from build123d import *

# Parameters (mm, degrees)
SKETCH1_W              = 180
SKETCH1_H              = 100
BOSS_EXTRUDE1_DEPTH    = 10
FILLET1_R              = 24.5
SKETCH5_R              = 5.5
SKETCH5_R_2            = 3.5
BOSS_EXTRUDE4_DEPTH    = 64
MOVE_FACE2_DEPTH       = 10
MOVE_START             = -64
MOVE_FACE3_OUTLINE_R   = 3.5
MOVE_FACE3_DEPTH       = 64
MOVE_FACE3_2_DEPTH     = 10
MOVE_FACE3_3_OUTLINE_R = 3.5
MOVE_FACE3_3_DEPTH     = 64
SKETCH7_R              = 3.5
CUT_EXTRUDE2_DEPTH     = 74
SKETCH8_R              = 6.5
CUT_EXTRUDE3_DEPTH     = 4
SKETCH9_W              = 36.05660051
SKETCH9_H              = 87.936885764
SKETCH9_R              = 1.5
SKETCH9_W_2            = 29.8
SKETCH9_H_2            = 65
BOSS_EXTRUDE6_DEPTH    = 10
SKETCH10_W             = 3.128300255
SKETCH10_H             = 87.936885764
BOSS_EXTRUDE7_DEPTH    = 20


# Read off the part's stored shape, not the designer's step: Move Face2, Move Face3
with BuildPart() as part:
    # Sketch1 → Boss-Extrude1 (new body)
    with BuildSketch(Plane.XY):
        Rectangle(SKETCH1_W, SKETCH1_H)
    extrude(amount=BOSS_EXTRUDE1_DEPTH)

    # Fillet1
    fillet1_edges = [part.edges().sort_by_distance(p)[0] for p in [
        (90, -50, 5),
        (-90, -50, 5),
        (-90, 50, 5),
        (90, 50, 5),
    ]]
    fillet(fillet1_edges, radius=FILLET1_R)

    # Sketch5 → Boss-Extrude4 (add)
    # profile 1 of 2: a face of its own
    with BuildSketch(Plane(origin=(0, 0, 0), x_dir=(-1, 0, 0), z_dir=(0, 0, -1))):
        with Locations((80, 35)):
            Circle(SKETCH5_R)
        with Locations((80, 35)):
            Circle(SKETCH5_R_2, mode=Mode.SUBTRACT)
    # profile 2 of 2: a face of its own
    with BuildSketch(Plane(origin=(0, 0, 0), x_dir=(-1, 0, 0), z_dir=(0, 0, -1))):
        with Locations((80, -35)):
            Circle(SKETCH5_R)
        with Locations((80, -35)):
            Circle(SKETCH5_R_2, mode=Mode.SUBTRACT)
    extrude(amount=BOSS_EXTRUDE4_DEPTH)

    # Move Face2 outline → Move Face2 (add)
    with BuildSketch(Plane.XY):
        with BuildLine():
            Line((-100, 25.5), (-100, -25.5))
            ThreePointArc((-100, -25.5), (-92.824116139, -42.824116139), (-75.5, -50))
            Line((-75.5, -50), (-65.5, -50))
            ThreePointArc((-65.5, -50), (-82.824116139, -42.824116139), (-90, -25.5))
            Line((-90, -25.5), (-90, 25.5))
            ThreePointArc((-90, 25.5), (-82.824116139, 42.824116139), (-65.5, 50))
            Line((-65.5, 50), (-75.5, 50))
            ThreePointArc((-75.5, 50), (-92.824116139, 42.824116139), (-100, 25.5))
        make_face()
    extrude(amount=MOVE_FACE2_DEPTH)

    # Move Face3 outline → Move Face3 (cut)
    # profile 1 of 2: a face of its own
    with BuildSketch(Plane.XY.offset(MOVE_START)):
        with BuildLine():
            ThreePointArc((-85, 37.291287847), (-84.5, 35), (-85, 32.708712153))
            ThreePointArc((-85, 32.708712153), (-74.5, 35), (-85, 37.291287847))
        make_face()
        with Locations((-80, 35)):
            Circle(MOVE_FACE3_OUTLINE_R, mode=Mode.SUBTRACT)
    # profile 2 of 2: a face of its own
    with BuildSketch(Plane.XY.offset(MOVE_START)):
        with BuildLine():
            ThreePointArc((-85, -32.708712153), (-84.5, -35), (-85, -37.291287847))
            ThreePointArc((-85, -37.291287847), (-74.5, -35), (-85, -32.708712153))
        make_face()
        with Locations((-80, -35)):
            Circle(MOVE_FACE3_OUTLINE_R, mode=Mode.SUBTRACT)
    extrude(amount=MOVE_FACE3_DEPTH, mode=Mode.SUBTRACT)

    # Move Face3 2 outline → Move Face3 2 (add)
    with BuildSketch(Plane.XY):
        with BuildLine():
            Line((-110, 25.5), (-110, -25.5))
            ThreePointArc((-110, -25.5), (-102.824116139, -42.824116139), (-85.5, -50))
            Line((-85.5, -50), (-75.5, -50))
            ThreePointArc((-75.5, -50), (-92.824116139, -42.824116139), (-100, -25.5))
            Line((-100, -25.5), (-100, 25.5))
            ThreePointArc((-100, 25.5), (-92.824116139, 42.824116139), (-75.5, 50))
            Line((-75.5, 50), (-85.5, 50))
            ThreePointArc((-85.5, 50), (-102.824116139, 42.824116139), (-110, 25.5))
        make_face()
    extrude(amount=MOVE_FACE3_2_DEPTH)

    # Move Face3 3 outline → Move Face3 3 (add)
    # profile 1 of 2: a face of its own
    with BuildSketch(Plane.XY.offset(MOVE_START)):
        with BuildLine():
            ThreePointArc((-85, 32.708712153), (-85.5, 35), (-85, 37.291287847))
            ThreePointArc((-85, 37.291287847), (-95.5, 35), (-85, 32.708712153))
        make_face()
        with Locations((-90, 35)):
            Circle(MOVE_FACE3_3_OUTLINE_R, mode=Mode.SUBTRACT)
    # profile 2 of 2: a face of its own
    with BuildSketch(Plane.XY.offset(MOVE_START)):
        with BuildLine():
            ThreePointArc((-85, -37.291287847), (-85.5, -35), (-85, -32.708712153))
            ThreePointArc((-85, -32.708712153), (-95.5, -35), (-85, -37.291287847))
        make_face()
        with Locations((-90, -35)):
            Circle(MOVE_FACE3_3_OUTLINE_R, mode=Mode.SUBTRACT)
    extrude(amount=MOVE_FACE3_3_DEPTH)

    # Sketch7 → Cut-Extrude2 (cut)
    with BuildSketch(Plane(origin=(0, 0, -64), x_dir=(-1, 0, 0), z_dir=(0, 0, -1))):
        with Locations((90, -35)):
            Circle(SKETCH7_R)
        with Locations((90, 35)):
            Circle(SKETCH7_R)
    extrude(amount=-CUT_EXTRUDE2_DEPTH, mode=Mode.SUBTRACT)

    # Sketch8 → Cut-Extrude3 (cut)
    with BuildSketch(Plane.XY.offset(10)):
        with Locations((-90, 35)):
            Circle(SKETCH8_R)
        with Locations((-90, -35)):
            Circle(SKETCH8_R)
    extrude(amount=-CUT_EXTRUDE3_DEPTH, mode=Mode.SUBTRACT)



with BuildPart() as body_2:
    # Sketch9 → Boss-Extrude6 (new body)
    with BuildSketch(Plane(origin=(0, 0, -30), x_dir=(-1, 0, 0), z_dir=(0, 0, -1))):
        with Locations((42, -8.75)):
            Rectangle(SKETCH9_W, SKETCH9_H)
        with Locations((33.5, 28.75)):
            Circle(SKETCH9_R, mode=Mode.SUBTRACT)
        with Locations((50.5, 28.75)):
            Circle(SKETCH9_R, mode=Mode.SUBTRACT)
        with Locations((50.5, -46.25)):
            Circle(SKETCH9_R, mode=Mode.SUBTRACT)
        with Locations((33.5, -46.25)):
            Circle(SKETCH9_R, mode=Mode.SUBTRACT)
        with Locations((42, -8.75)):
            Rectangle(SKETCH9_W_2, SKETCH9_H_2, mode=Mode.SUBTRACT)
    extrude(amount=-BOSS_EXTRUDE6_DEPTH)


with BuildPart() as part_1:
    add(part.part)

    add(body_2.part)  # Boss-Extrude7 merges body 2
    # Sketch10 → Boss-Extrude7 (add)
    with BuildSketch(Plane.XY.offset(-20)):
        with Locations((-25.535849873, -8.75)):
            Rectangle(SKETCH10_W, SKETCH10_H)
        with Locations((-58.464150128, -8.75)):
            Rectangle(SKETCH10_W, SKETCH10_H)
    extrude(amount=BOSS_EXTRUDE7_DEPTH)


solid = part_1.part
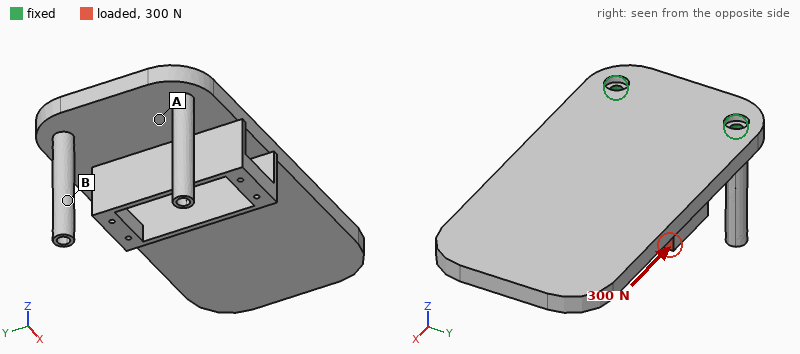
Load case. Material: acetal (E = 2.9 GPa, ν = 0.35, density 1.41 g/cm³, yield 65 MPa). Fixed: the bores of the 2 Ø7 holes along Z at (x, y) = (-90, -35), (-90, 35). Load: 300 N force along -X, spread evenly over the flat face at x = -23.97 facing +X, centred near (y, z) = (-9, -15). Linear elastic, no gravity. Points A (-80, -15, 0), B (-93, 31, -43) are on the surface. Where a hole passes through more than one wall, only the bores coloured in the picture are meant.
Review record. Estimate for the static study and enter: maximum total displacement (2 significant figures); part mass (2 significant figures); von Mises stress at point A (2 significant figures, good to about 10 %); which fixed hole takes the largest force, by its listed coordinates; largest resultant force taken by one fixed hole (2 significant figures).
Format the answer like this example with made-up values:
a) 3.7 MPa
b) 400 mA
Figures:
a) 2.5 mm
b) 320 g
c) 2.9 MPa
d) (-90, -35)
e) 190 N
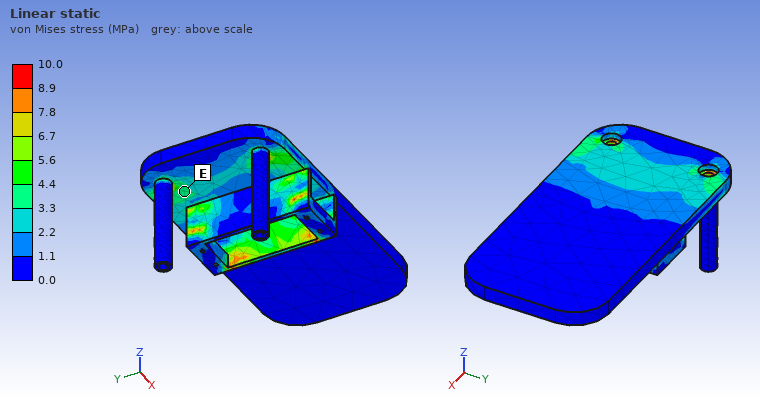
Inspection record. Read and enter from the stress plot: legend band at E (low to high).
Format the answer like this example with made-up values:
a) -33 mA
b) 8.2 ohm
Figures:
a) 3.3 to 4.4 MPa
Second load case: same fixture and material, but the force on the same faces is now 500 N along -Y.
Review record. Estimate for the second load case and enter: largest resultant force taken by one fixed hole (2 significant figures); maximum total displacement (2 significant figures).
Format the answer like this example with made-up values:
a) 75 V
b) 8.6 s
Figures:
a) 530 N
b) 0.75 mm
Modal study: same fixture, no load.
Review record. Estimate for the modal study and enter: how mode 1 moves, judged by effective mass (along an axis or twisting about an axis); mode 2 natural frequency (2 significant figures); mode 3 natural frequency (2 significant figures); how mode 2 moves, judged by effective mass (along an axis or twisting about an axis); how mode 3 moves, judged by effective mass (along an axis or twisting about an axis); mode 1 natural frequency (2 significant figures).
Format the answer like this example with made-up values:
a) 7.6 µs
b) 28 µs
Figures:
a) along Z
b) 270 Hz
c) 380 Hz
d) twisting about X
e) along Z
f) 63 Hz
